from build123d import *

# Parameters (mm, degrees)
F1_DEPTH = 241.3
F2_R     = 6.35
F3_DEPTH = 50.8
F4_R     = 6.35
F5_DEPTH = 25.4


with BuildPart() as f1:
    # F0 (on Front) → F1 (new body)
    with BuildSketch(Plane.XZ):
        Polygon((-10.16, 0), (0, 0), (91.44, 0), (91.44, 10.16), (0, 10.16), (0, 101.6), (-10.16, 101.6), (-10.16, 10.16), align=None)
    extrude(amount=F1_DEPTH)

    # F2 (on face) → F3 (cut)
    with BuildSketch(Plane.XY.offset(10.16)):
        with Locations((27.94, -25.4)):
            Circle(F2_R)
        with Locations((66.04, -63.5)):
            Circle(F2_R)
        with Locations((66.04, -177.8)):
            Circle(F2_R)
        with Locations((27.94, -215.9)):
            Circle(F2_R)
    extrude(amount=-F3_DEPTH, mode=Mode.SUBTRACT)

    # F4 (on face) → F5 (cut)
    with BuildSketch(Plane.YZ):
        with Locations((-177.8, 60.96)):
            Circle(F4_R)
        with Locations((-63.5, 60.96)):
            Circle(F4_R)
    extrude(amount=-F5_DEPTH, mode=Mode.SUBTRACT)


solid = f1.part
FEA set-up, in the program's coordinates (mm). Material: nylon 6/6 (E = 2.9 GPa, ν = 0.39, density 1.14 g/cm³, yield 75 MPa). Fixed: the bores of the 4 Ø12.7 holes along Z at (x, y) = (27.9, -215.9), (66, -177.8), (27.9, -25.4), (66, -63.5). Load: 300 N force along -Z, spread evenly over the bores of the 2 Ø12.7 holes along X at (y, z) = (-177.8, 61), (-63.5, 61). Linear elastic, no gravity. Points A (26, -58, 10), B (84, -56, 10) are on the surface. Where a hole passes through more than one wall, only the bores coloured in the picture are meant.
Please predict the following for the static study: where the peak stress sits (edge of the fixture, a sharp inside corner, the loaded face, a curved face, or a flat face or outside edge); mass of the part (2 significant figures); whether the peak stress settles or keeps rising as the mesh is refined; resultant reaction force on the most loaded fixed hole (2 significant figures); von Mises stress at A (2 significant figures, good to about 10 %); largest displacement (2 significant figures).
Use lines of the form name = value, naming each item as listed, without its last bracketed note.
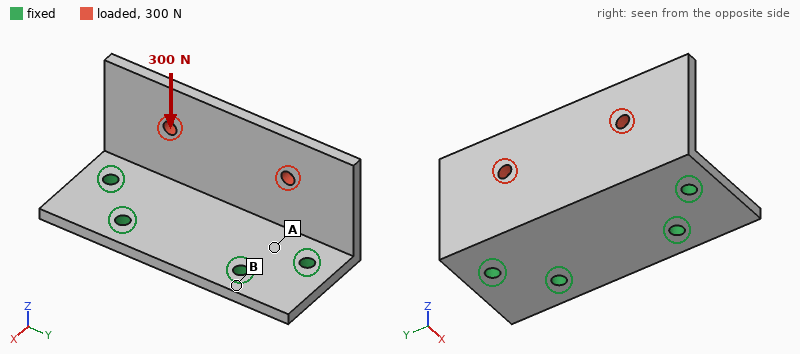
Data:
where the peak stress sits = edge of the fixture
mass of the part = 530 g
whether the peak stress settles or keeps rising as the mesh is refined = keeps rising
resultant reaction force on the most loaded fixed hole = 170 N
von Mises stress at A = 1.0 MPa
largest displacement = 0.34 mm
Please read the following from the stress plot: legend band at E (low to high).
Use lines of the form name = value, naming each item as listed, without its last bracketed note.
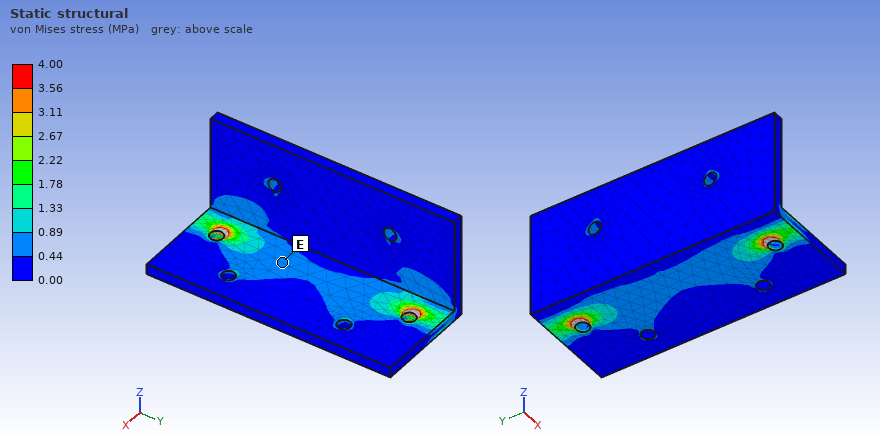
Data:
legend band at E = 0.44 to 0.89 MPa
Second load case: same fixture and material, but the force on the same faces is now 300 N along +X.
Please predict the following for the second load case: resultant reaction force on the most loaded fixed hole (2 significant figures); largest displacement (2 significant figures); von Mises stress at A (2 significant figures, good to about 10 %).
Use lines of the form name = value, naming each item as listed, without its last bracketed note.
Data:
resultant reaction force on the most loaded fixed hole = 160 N
largest displacement = 1.3 mm
von Mises stress at A = 2.5 MPa
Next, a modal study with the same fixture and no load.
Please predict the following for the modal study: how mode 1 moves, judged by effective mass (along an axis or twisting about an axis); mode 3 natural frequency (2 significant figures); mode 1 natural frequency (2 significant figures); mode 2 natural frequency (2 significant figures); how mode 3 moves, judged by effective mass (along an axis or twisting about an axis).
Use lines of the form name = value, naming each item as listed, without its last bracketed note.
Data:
how mode 1 moves, judged by effective mass = along X
mode 3 natural frequency = 560 Hz
mode 1 natural frequency = 190 Hz
mode 2 natural frequency = 300 Hz
how mode 3 moves, judged by effective mass = along Z
